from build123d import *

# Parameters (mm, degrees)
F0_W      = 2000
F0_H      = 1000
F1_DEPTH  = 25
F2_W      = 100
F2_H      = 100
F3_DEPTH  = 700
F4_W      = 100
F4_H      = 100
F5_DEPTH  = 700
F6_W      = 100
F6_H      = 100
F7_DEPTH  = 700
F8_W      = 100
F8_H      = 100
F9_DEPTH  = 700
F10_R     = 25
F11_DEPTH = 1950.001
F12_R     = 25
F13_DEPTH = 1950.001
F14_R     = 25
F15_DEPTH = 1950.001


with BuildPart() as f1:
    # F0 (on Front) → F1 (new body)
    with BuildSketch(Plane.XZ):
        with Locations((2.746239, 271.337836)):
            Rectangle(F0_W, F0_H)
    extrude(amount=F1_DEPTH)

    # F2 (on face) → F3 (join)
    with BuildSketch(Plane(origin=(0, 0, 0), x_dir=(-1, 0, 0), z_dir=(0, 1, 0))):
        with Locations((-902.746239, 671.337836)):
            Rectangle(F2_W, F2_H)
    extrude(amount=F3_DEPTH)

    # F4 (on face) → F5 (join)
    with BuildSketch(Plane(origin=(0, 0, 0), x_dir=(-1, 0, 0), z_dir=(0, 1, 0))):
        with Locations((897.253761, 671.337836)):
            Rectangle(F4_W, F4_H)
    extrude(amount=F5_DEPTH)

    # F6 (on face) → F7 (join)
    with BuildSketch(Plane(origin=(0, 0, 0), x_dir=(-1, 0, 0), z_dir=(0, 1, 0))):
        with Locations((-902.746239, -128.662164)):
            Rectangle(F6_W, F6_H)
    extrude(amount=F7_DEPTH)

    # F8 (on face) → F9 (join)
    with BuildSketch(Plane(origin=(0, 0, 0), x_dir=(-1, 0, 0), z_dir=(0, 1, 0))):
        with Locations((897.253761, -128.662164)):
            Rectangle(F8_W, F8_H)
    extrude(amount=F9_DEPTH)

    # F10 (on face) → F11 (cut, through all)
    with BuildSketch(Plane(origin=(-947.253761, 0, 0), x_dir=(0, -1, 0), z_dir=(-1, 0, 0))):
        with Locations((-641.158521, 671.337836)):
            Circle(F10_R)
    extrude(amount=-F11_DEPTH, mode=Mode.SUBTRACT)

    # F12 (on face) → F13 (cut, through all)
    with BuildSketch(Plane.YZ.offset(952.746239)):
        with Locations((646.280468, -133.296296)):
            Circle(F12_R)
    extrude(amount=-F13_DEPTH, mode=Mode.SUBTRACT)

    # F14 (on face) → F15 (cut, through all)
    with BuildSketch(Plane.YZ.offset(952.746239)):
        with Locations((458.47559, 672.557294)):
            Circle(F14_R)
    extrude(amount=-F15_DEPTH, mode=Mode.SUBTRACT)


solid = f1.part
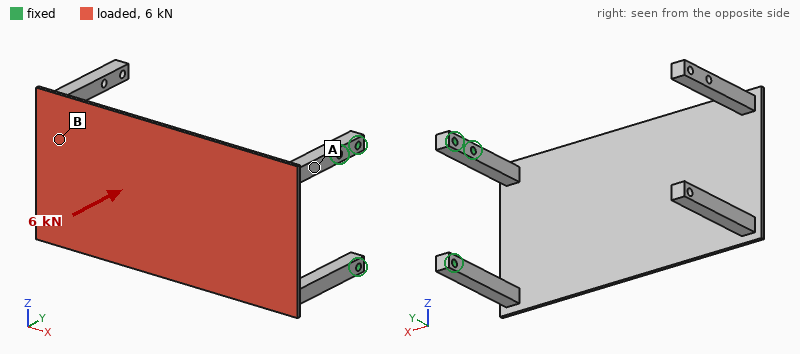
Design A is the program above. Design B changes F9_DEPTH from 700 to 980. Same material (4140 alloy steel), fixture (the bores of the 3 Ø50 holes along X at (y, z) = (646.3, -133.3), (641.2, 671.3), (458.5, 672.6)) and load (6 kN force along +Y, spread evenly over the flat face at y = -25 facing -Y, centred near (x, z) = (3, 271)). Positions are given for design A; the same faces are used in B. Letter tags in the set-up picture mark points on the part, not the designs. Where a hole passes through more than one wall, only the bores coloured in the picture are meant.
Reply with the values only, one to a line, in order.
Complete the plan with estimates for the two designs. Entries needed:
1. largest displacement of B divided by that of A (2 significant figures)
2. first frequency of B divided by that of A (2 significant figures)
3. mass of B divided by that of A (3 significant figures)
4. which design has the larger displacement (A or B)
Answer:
1.1
0.93
1.04
B
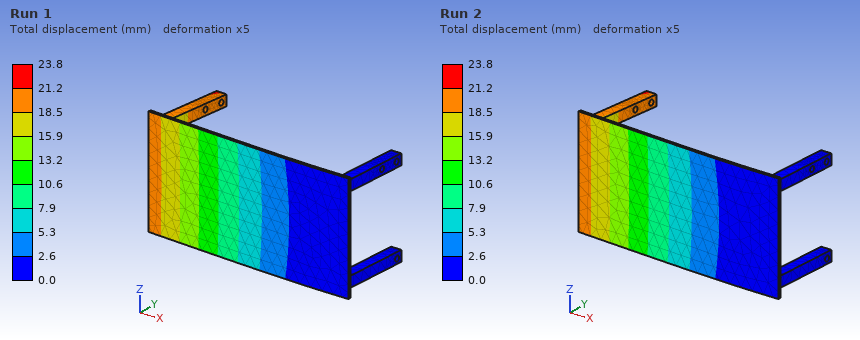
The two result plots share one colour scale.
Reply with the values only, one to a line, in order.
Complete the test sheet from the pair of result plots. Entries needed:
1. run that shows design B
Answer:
Run 2
